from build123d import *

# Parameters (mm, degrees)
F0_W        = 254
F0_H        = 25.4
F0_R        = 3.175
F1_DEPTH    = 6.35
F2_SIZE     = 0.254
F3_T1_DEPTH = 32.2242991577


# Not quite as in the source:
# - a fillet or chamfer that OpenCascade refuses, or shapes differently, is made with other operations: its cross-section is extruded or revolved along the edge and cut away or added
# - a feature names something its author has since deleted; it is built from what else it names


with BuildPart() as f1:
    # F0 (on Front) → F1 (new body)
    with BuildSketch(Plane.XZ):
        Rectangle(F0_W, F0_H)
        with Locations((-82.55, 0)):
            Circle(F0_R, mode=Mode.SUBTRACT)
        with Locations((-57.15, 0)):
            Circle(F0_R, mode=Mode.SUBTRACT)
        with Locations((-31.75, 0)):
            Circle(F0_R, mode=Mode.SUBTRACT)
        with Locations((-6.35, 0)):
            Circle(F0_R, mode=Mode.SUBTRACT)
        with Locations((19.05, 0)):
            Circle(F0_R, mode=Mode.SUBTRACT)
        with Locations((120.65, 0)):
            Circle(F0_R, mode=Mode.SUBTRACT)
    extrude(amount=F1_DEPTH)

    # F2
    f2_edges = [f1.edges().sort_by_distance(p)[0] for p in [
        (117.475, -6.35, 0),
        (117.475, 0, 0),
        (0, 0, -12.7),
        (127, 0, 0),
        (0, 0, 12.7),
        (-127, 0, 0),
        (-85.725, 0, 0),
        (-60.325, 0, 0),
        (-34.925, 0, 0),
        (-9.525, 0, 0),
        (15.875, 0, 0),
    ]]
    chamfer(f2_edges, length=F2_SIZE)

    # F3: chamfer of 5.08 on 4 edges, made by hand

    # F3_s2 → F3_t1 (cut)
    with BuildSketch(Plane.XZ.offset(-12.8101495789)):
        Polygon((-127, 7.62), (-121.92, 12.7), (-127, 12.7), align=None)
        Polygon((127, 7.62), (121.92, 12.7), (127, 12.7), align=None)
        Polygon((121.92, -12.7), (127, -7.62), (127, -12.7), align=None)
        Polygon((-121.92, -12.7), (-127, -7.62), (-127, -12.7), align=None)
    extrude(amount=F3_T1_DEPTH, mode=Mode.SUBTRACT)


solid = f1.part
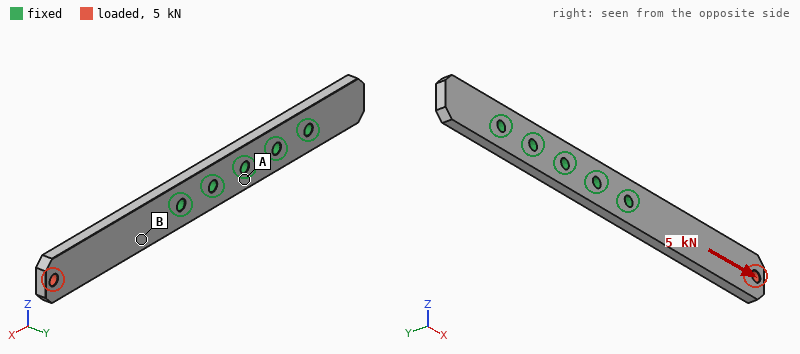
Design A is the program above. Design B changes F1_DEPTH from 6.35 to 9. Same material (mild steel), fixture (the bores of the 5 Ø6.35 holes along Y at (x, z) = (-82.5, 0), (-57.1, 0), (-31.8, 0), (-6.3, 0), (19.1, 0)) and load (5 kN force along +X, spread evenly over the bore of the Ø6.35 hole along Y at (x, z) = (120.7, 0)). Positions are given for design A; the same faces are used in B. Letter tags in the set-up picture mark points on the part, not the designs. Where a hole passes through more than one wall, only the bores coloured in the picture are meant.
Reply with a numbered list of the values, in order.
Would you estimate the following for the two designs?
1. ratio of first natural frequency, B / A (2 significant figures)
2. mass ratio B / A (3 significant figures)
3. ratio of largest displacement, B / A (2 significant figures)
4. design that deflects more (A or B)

1. 1.4
2. 1.42
3. 0.70
4. A
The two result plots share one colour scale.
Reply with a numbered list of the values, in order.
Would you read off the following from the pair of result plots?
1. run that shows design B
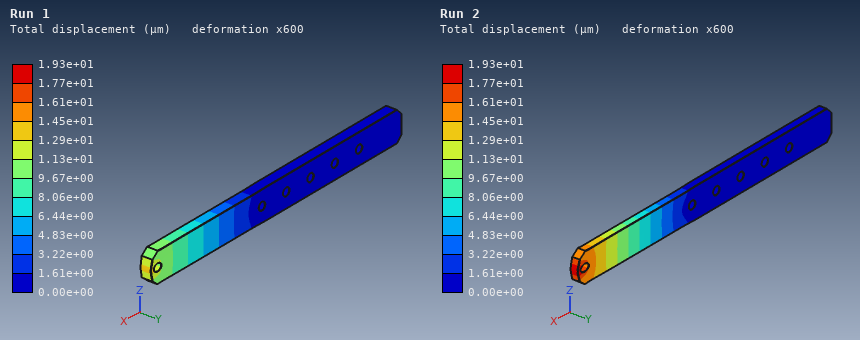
1. Run 1
